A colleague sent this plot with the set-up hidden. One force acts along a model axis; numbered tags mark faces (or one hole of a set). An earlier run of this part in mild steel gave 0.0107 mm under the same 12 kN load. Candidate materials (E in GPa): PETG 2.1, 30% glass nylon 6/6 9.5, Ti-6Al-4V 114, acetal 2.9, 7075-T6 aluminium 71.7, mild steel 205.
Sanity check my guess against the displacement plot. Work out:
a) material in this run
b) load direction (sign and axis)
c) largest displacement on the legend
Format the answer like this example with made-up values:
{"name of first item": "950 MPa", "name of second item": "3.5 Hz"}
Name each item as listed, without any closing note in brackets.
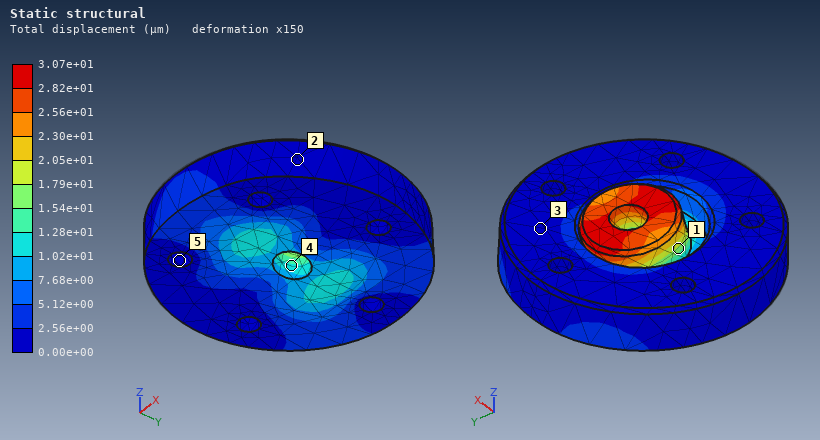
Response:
{"material in this run": "7075-T6 aluminium", "load direction": "+Y", "largest displacement on the legend": "3.07e+01 µm"}
